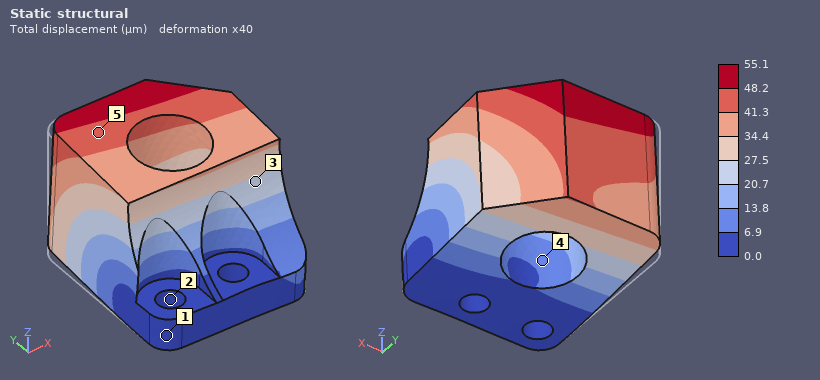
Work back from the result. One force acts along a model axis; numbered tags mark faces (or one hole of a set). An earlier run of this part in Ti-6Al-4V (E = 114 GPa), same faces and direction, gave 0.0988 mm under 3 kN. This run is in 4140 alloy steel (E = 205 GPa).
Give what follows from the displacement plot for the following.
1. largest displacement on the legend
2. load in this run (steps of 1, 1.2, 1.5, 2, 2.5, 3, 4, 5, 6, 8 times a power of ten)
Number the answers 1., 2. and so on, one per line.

1. 55.1 µm
2. 3 kN
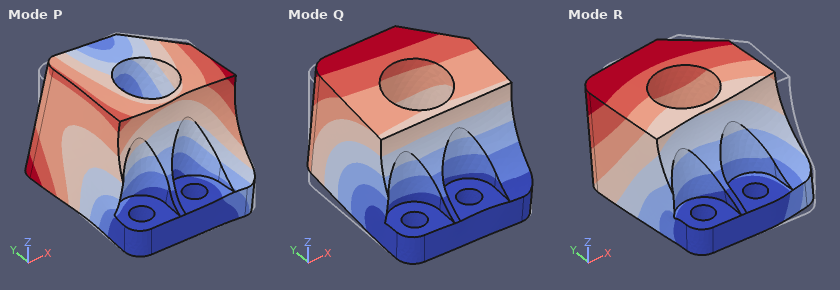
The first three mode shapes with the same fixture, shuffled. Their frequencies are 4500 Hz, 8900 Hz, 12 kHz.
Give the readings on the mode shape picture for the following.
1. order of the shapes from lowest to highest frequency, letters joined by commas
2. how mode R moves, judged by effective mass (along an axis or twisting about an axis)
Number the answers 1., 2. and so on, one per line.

1. Q, R, P
2. along X
